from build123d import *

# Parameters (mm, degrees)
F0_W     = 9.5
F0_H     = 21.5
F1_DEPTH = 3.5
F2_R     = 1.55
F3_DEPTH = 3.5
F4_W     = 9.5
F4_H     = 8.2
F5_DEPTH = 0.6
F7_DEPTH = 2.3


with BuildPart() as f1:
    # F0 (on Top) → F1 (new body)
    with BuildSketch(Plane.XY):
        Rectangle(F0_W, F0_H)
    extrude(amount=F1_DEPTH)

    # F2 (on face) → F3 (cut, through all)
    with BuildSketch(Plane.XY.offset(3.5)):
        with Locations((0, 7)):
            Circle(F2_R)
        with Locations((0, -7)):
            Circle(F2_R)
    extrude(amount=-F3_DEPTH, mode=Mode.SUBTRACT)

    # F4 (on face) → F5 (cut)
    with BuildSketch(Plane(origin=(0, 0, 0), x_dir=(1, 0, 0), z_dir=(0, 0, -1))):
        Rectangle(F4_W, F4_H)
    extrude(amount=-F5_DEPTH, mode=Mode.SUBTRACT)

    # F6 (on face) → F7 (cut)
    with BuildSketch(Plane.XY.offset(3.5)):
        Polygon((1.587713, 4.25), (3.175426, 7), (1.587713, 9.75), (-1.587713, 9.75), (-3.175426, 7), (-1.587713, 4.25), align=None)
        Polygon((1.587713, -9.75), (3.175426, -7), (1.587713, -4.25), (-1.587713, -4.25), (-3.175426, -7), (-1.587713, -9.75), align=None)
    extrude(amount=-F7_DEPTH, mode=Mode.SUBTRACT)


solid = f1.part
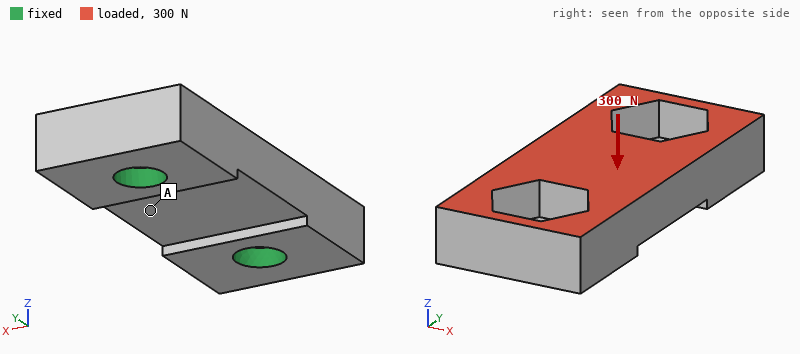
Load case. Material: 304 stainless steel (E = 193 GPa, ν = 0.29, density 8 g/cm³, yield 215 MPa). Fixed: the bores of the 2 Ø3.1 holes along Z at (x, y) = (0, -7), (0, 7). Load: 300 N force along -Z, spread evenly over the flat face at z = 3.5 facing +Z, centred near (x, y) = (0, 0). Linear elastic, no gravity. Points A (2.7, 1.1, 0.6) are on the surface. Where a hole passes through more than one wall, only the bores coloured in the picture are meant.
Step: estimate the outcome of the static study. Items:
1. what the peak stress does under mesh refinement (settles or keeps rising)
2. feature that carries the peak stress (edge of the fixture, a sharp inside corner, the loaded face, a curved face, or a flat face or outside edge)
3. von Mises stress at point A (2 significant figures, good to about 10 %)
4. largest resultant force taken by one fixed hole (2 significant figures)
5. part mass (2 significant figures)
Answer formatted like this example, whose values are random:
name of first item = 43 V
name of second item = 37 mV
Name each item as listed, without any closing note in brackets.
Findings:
what the peak stress does under mesh refinement = keeps rising
feature that carries the peak stress = edge of the fixture
von Mises stress at point A = 6.3 MPa
largest resultant force taken by one fixed hole = 170 N
part mass = 4.2 g
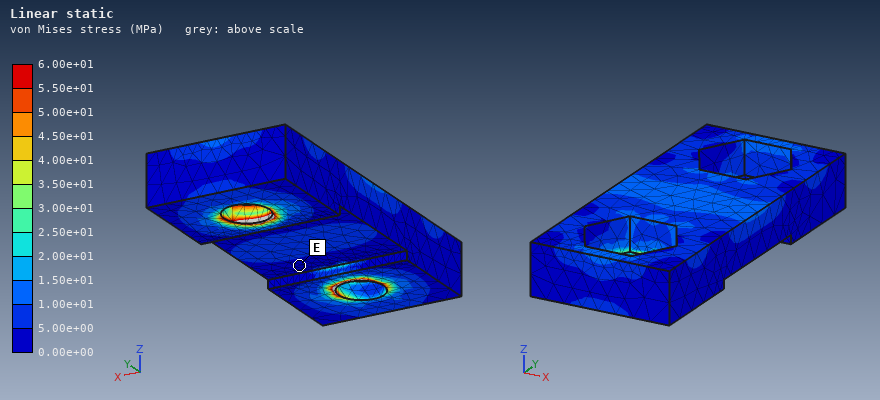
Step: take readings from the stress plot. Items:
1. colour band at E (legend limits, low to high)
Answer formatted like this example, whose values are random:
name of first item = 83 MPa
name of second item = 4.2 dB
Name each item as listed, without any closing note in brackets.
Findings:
colour band at E = 0.00e+00 to 5.00e+00 MPa
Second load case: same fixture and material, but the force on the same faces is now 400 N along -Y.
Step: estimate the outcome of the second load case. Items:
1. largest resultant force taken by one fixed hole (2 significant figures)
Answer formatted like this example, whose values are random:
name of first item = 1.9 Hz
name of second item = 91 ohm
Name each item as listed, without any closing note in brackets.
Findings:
largest resultant force taken by one fixed hole = 210 N
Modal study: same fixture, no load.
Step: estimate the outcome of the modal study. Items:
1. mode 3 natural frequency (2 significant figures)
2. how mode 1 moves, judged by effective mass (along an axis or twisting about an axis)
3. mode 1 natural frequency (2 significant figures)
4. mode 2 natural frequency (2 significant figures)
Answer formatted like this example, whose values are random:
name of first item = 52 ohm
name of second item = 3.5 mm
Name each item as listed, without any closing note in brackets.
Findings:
mode 3 natural frequency = 49 kHz
how mode 1 moves, judged by effective mass = along X
mode 1 natural frequency = 30 kHz
mode 2 natural frequency = 47 kHz
